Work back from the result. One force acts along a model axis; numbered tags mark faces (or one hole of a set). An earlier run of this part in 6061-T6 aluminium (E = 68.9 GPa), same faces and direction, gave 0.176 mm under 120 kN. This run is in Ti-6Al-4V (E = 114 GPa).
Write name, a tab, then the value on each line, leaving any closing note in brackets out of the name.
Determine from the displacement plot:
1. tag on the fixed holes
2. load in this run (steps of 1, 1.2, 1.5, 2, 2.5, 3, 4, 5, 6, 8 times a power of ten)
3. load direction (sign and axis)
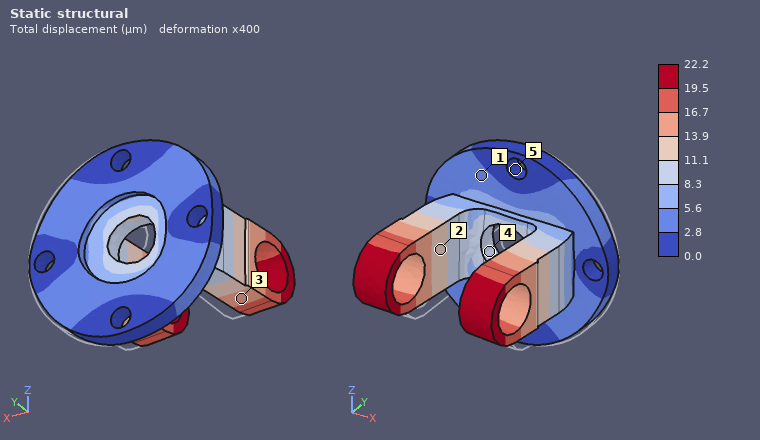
tag on the fixed holes	5
load in this run	25 kN
load direction	-X
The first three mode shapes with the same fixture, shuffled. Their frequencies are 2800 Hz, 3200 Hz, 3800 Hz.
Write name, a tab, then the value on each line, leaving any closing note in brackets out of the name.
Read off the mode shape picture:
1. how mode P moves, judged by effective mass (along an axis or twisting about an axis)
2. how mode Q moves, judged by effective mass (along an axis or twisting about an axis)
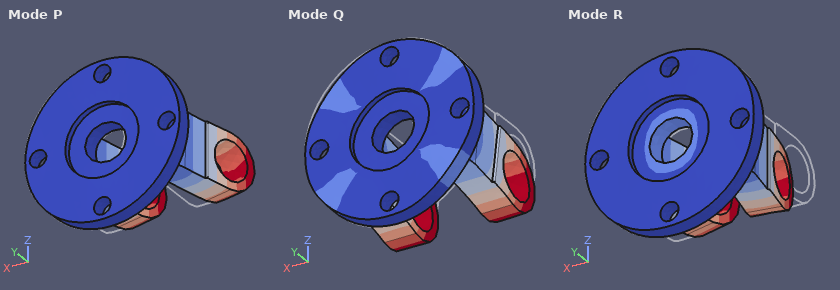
how mode P moves, judged by effective mass	along X
how mode Q moves, judged by effective mass	along Z
